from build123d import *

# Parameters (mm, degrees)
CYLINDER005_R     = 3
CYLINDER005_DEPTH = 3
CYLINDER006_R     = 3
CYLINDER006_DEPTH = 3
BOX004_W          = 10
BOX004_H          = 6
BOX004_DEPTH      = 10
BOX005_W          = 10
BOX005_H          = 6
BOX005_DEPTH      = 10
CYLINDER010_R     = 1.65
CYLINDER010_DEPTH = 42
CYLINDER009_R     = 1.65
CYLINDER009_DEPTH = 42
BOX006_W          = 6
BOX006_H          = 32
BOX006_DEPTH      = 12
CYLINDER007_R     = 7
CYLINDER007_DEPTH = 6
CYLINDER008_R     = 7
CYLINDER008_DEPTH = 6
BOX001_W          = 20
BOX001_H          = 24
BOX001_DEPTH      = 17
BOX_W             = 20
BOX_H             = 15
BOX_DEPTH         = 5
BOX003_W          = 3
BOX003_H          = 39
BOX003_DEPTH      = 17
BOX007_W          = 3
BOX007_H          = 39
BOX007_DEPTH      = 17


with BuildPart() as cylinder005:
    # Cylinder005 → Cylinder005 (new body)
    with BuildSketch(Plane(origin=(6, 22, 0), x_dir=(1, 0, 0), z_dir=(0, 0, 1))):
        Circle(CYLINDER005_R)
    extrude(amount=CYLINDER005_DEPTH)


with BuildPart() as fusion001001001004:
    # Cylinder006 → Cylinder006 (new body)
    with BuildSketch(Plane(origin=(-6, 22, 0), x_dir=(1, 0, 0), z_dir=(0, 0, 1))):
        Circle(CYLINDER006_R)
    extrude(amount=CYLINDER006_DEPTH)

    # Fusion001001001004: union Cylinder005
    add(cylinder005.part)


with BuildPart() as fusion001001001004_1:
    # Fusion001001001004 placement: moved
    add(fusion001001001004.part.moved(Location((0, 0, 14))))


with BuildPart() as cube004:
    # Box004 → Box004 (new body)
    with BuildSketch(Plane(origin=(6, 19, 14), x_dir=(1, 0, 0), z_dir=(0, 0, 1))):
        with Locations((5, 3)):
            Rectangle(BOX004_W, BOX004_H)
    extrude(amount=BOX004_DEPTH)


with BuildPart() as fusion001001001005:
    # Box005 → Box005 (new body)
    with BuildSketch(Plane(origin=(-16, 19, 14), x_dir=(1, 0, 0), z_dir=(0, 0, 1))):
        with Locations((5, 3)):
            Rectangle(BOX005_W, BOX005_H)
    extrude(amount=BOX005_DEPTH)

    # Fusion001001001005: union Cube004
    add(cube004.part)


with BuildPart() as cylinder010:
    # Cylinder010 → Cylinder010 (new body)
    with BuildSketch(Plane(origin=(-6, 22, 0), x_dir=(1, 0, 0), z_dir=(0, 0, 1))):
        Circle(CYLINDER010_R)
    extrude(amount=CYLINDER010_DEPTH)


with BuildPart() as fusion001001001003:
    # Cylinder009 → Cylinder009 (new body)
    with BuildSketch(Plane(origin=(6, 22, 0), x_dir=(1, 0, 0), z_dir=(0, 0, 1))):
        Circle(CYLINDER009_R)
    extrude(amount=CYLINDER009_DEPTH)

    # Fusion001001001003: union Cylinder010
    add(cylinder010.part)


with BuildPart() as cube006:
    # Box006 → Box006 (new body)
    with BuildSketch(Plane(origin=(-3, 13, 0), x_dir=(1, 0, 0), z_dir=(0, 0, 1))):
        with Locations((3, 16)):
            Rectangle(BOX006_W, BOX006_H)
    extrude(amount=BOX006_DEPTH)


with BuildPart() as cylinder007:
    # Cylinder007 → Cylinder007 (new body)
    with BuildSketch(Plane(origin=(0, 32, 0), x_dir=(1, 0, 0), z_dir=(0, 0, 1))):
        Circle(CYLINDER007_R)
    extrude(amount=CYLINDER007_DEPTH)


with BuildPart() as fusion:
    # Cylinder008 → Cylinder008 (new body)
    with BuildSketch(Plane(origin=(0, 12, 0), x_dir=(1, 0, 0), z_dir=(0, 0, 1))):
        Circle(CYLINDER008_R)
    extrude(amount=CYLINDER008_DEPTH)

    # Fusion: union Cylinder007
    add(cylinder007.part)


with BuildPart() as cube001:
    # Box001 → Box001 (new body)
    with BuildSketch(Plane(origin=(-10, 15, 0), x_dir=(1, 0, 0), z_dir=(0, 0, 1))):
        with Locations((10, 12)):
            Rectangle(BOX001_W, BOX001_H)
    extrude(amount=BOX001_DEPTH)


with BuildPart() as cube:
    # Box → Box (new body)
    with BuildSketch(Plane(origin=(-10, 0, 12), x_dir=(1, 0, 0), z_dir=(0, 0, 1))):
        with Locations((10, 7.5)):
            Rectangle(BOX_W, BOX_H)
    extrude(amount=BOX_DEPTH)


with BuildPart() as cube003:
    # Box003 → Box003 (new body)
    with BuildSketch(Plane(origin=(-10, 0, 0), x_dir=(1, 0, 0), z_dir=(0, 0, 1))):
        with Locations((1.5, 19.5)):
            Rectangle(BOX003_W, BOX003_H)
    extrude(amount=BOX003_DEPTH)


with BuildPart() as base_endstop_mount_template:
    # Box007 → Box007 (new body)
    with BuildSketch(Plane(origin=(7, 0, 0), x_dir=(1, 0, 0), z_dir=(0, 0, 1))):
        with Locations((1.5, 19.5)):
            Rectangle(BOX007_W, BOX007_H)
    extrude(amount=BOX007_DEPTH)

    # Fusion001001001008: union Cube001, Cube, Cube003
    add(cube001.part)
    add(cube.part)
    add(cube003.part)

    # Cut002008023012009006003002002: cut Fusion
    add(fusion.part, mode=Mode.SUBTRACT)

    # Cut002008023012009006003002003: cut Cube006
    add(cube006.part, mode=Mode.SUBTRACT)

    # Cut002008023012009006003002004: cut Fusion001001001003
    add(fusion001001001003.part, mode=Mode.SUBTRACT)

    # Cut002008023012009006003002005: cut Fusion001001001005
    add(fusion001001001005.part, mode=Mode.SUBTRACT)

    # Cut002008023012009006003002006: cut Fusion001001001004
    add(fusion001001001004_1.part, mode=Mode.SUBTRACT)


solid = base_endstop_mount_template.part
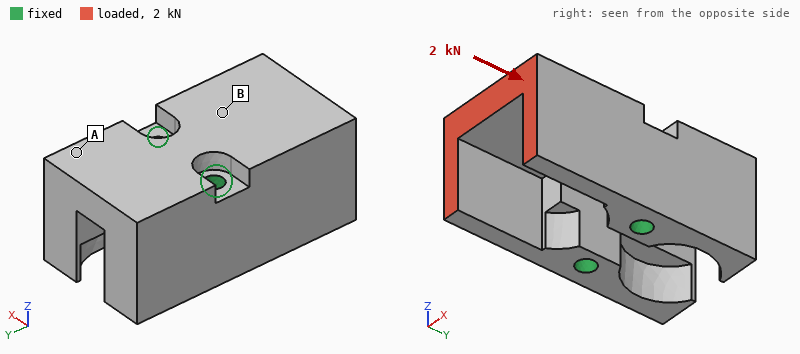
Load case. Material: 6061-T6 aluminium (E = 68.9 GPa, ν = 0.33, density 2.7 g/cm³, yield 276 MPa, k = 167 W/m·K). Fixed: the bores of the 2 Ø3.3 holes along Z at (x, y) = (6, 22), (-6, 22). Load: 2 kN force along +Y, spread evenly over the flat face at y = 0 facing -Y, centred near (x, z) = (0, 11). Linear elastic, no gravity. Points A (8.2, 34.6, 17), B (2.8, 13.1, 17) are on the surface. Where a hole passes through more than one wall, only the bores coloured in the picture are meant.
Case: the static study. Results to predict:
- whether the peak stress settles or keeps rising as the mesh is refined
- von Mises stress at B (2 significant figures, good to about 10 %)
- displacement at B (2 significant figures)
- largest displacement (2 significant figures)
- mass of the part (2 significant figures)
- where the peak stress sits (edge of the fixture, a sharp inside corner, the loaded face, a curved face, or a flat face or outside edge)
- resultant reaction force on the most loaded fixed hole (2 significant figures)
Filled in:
keeps rising
10 MPa
3.3 µm
6.0 µm
22 g
edge of the fixture
1.0 kN
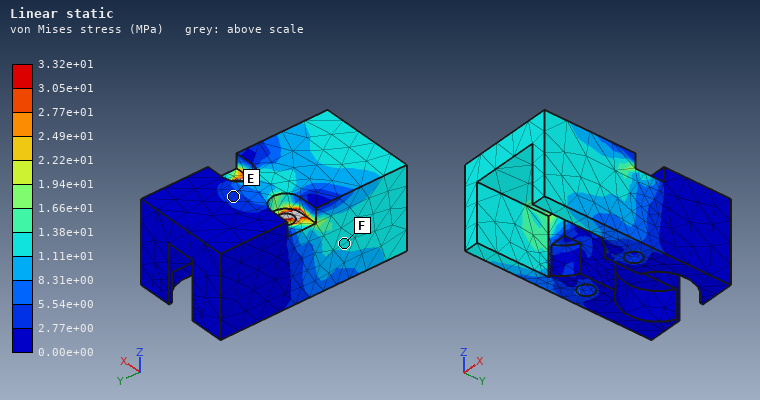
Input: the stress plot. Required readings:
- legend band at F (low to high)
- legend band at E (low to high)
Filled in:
1.11e+01 to 1.38e+01 MPa
2.77e+00 to 5.54e+00 MPa
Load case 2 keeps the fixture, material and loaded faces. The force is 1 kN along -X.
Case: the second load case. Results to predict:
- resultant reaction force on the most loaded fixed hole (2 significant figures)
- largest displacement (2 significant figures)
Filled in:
1.3 kN
71 µm
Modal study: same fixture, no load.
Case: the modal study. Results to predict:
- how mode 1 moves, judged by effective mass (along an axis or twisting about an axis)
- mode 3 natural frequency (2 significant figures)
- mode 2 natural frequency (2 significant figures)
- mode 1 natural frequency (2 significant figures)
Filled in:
along X
19 kHz
17 kHz
15 kHz
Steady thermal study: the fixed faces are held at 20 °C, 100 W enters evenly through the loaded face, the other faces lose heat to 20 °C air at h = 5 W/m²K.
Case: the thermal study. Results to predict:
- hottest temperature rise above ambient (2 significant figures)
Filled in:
73 K
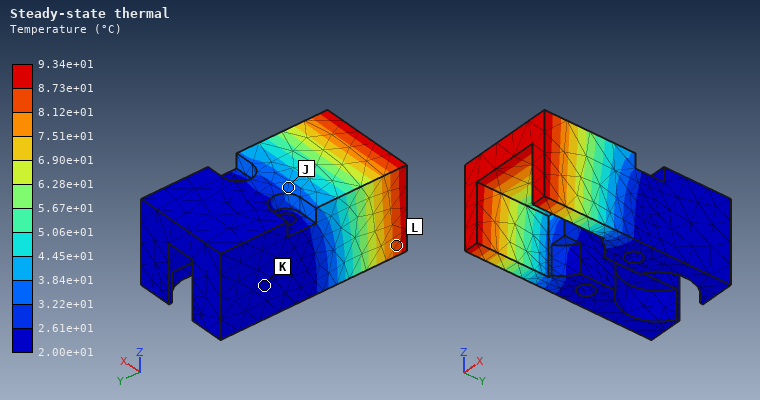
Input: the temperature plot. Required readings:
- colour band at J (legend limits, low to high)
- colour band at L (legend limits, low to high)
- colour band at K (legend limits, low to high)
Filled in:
3.22e+01 to 3.84e+01 °C
8.12e+01 to 8.73e+01 °C
2.00e+01 to 2.61e+01 °C
